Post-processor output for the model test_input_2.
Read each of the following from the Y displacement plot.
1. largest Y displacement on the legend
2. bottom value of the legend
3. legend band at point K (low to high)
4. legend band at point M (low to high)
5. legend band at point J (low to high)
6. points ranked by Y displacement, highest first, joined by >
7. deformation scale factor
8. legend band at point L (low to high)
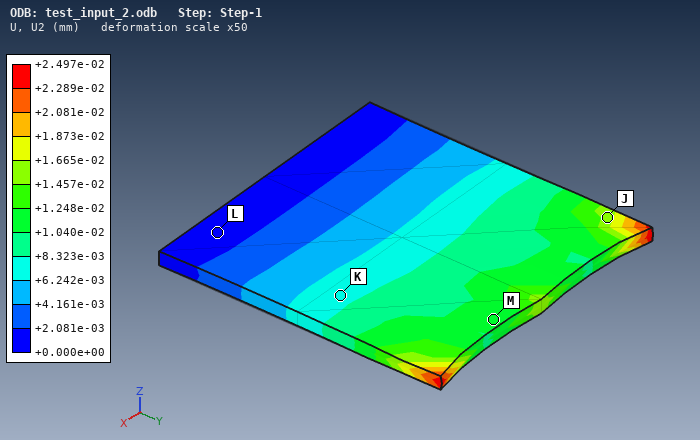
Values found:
+2.497e-02 mm
+0.000e+00 mm
+6.242e-03 to +8.323e-03 mm
+1.040e-02 to +1.248e-02 mm
+1.457e-02 to +1.665e-02 mm
J > M > K > L
50
+0.000e+00 to +2.081e-03 mm
